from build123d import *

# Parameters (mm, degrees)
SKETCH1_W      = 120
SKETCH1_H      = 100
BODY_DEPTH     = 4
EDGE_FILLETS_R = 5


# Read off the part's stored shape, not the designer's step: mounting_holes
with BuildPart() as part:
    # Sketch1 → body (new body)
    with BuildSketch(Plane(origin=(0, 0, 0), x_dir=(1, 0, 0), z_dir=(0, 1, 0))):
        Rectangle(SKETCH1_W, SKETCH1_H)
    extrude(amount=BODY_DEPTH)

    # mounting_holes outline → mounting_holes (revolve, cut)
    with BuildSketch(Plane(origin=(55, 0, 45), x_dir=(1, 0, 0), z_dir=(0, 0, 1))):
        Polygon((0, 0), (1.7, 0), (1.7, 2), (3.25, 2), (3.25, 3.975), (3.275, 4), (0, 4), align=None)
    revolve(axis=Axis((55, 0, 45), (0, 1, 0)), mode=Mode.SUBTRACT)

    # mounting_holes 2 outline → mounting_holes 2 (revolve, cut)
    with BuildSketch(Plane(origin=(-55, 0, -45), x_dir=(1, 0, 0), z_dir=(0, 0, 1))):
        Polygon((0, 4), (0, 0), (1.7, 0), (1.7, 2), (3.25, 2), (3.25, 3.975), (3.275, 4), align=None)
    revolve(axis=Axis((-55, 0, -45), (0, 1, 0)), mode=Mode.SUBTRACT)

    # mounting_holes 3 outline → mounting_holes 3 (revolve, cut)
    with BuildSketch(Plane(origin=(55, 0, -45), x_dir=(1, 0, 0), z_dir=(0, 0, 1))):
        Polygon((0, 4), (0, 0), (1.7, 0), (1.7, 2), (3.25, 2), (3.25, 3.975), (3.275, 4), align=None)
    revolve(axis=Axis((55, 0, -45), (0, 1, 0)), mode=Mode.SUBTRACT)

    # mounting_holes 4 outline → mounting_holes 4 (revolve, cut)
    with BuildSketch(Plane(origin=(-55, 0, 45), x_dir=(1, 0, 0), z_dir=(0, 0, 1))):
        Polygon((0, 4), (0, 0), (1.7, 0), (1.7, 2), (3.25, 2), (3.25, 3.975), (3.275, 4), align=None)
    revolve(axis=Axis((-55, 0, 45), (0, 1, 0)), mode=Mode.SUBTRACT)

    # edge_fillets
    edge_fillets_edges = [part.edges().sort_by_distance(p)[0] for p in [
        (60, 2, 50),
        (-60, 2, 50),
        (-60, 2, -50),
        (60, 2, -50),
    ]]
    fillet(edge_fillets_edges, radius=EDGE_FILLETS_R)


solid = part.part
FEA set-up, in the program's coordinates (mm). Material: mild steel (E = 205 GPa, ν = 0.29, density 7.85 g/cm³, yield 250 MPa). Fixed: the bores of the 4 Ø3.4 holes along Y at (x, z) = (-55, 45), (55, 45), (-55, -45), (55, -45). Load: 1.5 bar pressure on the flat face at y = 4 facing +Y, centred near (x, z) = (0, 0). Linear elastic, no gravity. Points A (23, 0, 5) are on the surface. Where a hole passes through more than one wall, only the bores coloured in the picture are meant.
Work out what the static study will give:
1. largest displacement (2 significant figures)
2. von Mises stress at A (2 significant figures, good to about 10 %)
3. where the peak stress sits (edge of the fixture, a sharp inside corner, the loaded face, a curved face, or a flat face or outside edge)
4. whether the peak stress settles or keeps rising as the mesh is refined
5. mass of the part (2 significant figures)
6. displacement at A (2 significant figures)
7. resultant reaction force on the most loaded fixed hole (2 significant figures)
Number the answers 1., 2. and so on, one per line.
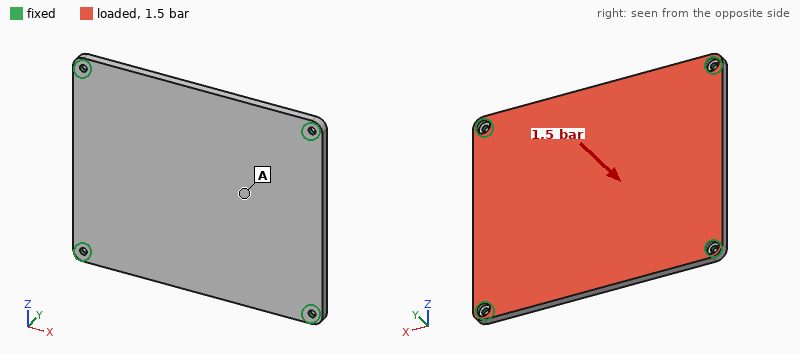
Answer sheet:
1. 0.16 mm
2. 32 MPa
3. edge of the fixture
4. keeps rising
5. 370 g
6. 0.14 mm
7. 1.0 kN
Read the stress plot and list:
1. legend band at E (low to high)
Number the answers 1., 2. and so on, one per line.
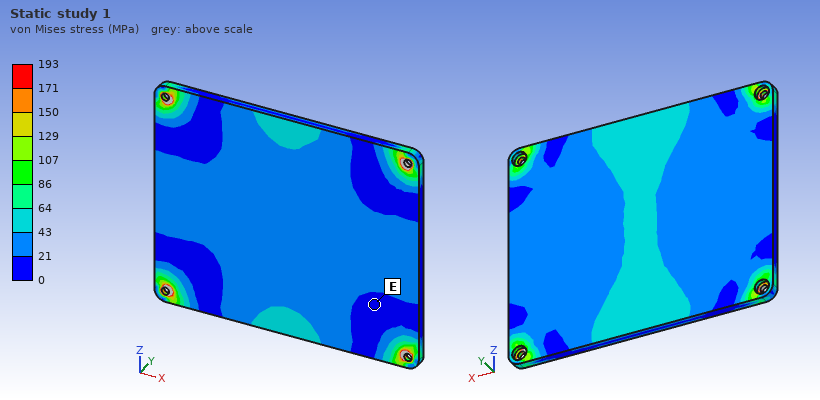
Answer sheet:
1. 0 to 21 MPa
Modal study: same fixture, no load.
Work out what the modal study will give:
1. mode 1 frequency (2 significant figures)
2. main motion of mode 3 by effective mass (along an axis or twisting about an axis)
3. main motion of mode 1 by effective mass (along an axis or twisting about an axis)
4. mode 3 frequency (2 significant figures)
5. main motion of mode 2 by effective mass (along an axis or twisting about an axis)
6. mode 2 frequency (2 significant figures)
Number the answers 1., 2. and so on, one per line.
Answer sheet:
1. 1000 Hz
2. twisting about Z
3. along Y
4. 2200 Hz
5. twisting about X
6. 1800 Hz
